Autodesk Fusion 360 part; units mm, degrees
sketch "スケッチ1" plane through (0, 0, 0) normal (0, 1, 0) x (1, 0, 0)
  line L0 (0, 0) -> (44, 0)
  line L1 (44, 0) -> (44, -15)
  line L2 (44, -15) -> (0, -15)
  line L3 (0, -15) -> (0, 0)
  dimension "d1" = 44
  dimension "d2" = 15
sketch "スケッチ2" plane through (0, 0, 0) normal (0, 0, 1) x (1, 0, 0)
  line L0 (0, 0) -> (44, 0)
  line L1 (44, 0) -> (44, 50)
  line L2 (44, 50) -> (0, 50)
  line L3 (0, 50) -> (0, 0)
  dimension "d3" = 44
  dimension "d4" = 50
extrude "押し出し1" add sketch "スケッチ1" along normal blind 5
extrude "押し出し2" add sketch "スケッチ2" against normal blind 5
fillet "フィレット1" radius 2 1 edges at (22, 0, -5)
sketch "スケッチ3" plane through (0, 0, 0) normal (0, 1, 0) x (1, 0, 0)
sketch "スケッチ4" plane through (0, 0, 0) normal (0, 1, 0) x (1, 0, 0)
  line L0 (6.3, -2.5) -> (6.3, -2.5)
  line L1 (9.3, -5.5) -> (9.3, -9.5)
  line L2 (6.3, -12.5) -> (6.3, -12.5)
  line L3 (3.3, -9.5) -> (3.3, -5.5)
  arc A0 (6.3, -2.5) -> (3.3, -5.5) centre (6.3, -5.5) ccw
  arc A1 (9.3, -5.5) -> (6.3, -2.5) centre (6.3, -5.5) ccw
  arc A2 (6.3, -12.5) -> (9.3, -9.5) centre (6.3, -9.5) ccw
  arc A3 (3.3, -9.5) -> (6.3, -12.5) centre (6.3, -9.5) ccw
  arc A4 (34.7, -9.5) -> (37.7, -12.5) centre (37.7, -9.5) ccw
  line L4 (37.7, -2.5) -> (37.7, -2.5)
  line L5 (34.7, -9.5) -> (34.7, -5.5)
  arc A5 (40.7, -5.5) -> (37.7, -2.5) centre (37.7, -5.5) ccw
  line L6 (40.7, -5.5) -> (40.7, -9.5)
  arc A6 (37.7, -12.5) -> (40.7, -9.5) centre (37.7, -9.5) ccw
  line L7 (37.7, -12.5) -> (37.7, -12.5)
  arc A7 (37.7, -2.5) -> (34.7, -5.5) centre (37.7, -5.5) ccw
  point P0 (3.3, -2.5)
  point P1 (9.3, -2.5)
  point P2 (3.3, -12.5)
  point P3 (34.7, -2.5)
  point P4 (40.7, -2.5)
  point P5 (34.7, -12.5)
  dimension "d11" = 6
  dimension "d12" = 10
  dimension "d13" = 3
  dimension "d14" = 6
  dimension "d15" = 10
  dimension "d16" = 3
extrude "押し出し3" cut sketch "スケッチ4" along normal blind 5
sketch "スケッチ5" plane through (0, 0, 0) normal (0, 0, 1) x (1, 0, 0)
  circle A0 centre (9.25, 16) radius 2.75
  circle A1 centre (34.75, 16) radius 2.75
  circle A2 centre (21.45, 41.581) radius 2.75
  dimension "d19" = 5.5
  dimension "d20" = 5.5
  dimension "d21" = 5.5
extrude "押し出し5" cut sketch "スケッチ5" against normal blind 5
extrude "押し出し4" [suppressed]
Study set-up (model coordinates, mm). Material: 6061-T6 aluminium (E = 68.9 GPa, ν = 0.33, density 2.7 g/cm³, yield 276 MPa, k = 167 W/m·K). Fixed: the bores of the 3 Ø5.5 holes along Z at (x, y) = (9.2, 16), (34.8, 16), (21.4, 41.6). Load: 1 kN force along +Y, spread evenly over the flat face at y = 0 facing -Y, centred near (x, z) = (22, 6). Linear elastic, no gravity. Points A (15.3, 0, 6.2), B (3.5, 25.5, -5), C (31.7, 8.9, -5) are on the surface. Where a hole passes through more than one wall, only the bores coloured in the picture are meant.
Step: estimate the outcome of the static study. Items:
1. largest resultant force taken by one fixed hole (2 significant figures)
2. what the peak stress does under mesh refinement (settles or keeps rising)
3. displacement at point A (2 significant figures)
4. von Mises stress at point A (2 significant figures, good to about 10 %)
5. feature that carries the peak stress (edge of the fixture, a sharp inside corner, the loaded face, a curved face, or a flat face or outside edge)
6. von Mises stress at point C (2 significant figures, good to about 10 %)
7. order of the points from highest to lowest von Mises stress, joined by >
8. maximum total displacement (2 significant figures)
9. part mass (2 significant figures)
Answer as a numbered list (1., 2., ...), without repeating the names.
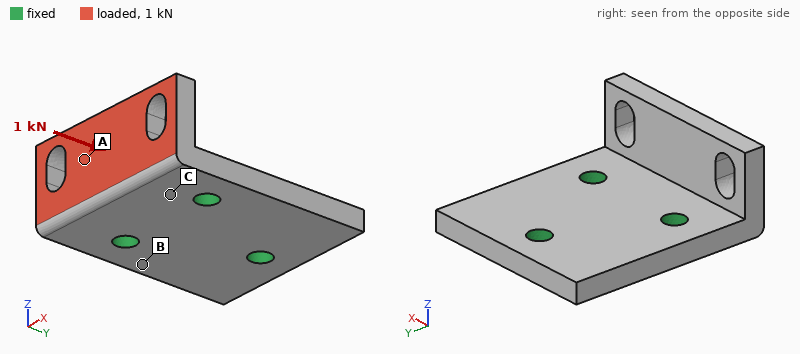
1. 460 N
2. keeps rising
3. 46 µm
4. 14 MPa
5. edge of the fixture
6. 38 MPa
7. C > A > B
8. 79 µm
9. 36 g
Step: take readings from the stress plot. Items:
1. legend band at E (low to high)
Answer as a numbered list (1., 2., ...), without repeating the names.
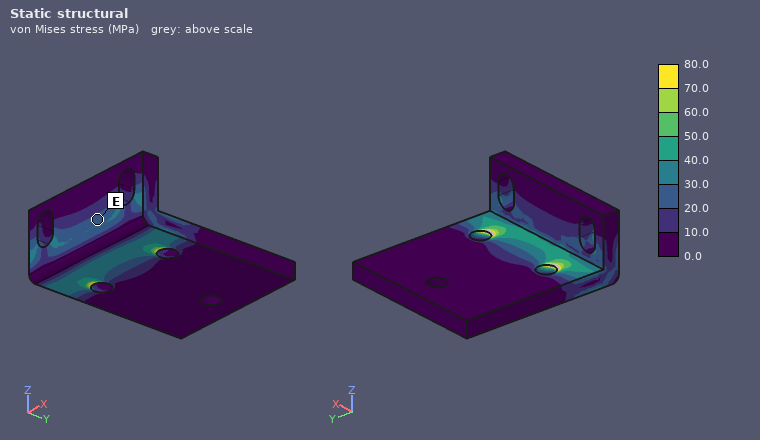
1. 20.0 to 30.0 MPa
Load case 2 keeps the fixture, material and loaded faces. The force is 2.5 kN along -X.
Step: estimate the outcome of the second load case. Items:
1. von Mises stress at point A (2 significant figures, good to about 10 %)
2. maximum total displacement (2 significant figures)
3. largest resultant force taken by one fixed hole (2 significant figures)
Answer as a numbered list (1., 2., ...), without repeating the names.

1. 14 MPa
2. 45 µm
3. 1.9 kN
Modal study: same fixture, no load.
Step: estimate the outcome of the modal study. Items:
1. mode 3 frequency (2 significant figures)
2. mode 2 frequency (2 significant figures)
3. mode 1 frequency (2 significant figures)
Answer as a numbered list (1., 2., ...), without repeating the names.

1. 11 kHz
2. 9900 Hz
3. 6300 Hz
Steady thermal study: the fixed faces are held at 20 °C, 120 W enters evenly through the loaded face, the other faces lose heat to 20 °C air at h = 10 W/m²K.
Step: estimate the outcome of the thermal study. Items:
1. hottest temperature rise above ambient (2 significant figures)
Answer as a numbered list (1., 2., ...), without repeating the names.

1. 74 K
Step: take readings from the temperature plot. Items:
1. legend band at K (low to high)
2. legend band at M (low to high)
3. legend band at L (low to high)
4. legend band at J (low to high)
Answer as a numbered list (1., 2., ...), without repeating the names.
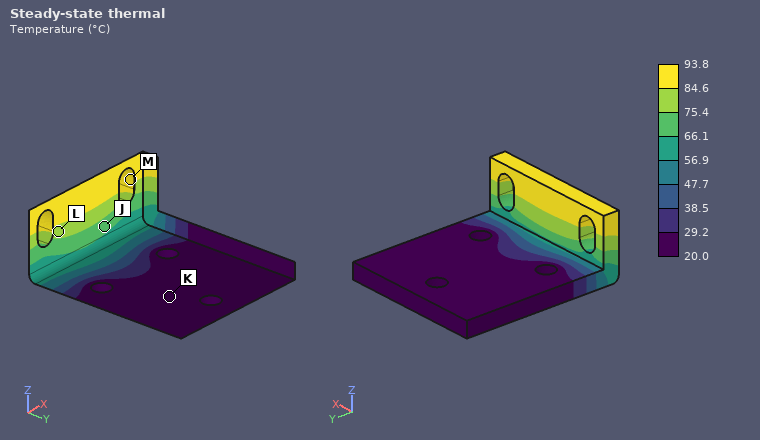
1. 20.0 to 29.2 °C
2. 84.6 to 93.8 °C
3. 75.4 to 84.6 °C
4. 66.1 to 75.4 °C
